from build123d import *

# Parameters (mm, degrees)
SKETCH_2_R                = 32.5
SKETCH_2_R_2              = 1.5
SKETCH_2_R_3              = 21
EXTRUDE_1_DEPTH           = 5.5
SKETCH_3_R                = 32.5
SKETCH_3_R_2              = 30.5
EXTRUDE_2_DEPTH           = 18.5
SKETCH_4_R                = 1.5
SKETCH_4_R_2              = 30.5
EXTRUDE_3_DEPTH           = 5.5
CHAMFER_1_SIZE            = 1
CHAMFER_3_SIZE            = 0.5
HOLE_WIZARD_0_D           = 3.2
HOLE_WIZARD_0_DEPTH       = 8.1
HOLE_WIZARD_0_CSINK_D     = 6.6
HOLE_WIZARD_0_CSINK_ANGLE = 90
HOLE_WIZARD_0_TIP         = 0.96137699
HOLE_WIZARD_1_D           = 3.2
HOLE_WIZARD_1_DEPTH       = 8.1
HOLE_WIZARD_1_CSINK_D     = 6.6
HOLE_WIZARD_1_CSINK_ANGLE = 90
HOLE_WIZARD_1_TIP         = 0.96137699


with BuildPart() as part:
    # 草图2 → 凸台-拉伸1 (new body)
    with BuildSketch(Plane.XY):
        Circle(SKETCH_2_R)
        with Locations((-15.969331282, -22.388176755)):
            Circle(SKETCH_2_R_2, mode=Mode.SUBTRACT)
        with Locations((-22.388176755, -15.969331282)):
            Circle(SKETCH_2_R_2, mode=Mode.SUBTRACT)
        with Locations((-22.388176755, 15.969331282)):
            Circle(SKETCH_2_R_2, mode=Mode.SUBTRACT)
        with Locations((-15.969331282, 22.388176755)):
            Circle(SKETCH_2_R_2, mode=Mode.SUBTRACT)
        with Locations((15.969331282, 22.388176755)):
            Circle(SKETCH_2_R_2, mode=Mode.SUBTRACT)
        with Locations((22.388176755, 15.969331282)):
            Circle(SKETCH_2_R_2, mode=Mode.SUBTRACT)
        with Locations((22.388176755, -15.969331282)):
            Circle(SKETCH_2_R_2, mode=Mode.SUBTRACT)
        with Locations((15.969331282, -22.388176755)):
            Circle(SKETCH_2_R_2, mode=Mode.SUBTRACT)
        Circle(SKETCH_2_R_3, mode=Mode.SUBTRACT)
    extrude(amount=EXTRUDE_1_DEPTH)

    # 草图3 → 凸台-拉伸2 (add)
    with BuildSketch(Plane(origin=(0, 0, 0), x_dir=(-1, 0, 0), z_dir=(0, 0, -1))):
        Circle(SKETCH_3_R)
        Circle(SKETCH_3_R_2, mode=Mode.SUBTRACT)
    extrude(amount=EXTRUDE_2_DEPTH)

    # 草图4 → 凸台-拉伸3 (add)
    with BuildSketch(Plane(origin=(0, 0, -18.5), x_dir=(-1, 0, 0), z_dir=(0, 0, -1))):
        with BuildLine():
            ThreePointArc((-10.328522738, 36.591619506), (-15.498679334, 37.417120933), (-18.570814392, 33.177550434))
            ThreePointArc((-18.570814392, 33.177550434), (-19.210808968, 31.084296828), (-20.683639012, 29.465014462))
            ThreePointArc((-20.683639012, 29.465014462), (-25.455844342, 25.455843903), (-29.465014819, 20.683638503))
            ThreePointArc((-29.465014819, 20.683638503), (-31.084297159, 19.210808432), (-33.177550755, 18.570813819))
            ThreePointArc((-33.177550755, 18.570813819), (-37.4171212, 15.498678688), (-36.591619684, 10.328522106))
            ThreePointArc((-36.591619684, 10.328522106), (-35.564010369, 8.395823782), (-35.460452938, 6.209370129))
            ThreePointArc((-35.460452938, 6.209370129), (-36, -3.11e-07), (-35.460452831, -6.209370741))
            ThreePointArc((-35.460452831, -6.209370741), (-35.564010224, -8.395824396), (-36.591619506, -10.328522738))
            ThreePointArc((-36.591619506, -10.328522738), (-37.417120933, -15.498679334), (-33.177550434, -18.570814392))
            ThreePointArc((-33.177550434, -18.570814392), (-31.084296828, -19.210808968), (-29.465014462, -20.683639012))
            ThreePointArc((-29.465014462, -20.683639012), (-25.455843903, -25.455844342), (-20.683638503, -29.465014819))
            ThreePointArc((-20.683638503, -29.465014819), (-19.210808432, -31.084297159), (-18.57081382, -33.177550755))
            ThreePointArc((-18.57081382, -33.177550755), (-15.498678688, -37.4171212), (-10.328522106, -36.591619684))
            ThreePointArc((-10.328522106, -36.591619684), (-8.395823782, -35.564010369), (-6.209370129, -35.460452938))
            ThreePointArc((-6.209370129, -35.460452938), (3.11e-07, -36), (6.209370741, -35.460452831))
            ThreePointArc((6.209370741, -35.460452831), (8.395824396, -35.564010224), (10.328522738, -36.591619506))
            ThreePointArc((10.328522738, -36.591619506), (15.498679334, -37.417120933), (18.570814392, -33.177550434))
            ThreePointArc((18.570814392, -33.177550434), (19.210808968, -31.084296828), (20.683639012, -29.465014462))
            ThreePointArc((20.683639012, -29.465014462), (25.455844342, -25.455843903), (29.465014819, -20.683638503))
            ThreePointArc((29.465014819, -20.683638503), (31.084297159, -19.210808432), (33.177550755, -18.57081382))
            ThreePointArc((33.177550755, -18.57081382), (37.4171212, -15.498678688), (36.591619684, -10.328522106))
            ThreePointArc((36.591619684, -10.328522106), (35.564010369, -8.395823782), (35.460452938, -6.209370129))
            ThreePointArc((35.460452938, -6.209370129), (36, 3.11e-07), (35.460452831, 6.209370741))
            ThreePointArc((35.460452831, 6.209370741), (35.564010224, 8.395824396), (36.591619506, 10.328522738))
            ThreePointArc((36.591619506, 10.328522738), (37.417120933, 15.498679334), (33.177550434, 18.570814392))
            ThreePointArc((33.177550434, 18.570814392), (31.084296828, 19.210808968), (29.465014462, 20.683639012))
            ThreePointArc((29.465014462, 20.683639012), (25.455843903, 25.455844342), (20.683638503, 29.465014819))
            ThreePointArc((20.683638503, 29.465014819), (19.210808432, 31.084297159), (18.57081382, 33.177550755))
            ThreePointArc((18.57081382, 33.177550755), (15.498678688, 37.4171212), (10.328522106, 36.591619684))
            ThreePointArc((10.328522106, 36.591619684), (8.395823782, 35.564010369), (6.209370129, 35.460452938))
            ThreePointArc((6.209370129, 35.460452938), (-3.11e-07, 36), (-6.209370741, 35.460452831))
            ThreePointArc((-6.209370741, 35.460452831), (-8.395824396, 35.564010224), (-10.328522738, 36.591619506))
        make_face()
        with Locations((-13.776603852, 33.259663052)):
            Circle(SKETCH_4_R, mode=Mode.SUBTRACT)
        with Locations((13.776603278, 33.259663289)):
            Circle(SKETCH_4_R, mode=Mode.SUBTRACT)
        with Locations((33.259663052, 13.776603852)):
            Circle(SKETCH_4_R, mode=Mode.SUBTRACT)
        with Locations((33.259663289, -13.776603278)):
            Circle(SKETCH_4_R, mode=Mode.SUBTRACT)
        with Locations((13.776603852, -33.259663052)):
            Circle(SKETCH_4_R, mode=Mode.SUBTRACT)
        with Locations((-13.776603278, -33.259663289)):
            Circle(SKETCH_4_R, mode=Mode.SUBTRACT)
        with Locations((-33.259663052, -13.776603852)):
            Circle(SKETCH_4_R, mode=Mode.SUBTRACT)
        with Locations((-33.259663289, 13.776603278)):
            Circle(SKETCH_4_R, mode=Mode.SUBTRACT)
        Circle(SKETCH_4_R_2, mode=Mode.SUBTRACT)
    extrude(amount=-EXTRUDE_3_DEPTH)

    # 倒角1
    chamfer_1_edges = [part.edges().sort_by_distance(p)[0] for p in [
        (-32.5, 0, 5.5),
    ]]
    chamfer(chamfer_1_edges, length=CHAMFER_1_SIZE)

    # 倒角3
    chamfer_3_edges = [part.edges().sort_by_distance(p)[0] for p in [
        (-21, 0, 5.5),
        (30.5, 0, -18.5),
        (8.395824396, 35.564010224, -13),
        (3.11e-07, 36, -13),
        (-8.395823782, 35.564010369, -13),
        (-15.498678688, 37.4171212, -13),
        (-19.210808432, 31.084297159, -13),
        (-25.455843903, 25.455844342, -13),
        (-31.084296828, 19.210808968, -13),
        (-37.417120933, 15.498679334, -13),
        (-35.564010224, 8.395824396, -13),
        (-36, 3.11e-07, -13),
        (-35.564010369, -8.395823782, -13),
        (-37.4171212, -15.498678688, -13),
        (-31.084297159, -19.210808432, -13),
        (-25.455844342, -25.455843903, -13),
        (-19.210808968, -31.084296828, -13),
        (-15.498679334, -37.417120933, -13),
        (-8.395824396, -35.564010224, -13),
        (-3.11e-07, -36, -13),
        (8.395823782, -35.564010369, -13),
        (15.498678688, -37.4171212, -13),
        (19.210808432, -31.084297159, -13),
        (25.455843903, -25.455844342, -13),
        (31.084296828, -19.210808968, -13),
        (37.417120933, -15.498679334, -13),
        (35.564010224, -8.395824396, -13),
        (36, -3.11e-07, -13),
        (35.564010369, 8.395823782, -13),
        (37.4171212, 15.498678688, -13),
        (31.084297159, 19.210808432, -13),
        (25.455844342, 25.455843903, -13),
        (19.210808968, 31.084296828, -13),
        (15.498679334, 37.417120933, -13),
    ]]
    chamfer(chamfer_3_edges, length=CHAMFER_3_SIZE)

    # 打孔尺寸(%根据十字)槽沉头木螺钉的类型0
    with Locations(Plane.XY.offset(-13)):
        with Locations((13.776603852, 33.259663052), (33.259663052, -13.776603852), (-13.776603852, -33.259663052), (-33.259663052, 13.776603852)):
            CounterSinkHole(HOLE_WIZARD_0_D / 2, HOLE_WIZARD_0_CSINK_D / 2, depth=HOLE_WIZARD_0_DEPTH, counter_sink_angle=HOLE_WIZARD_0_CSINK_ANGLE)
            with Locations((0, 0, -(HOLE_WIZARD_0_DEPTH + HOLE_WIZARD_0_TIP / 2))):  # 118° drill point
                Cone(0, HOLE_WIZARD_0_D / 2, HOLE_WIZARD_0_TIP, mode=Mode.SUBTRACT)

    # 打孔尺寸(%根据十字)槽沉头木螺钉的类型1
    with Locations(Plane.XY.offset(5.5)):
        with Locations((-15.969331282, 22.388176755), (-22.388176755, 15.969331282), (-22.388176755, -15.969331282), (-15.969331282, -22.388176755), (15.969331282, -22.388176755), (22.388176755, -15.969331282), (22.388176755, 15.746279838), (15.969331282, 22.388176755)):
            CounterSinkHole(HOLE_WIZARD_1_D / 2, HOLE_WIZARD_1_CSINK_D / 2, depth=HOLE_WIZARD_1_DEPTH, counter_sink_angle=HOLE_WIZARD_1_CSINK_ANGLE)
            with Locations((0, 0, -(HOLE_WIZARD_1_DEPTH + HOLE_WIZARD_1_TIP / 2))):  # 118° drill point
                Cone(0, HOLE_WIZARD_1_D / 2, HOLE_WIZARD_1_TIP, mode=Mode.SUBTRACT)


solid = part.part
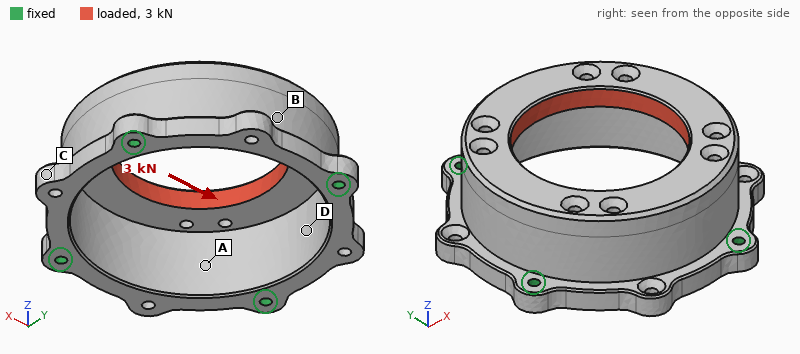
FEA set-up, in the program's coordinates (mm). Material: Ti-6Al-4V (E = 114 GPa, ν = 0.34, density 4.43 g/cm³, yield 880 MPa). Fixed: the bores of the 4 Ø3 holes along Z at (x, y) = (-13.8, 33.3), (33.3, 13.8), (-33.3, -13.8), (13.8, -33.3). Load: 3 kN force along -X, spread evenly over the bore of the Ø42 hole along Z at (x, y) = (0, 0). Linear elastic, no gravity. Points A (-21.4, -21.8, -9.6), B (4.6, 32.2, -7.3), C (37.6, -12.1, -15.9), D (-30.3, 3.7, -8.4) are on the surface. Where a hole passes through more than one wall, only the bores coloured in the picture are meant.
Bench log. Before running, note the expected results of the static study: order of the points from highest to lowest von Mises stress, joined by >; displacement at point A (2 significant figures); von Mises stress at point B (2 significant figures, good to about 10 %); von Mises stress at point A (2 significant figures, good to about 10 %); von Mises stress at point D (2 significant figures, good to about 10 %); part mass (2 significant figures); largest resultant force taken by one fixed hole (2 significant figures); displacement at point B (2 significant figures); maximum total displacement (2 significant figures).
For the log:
A > B > D > C
4.2 µm
22 MPa
31 MPa
15 MPa
100 g
1.0 kN
5.5 µm
15 µm
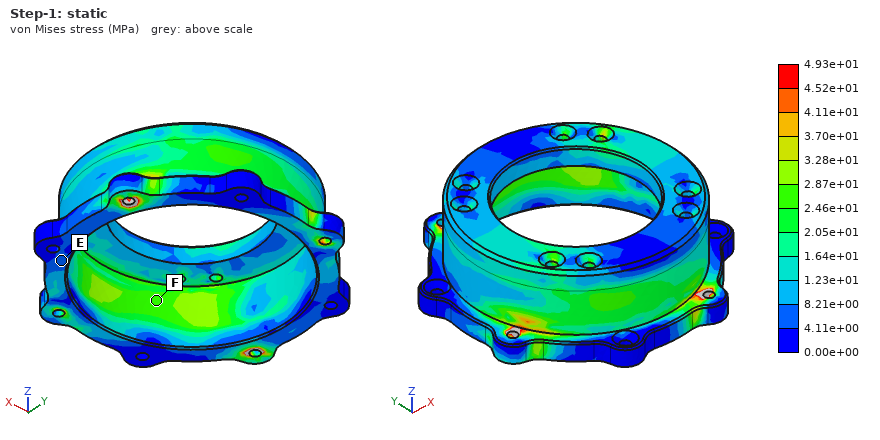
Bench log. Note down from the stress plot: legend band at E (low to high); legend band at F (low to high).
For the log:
4.11e+00 to 8.21e+00 MPa
2.46e+01 to 2.87e+01 MPa
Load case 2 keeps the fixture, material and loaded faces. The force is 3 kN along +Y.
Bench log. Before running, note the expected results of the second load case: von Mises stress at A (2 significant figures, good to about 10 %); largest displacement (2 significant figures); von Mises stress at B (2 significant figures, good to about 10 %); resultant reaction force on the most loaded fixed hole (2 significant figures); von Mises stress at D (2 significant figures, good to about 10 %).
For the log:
12 MPa
15 µm
9.1 MPa
1.0 kN
28 MPa
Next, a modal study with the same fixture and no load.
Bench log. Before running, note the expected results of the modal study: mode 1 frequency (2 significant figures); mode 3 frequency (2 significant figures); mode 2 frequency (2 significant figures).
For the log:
9400 Hz
10000 Hz
10000 Hz
